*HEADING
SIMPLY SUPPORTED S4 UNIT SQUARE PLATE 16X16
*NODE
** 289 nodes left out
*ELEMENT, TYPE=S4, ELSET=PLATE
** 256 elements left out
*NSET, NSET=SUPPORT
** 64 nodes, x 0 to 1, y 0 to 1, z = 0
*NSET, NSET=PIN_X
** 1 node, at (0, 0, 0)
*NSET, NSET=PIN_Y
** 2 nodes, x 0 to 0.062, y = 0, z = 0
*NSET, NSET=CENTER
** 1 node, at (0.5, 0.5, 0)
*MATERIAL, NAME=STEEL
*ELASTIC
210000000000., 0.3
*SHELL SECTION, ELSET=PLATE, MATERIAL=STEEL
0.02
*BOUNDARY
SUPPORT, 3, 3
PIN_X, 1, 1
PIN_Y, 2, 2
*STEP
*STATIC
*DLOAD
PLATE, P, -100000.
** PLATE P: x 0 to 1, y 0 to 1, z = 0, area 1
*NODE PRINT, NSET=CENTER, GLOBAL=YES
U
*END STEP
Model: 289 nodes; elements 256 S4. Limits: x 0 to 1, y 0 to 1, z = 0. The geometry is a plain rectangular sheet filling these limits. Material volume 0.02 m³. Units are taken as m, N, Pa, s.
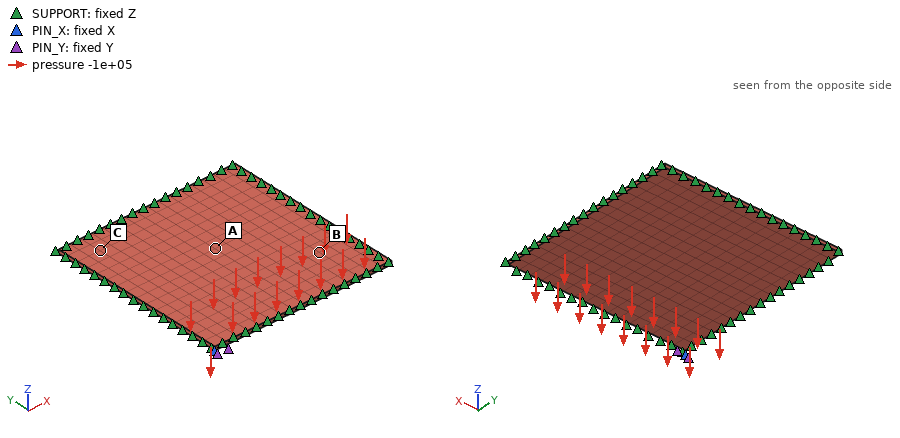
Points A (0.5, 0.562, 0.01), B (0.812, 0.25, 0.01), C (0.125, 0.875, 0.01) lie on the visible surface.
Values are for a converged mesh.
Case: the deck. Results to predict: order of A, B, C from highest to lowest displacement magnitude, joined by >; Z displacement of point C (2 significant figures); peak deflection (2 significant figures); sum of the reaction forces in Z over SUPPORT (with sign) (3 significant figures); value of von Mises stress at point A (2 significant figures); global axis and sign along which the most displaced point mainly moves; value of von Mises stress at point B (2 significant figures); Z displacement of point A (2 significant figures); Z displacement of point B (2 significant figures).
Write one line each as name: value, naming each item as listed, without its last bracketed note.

order of A, B, C from highest to lowest displacement magnitude, joined by >: A > B > C
Z displacement of point C: -4.4e-04 m
peak deflection: 0.0027 m
sum of the reaction forces in Z over SUPPORT (with sign): 1.00e+05 N
value of von Mises stress at point A: 7.2e+07 Pa
global axis and sign along which the most displaced point mainly moves: -Z
value of von Mises stress at point B: 5.7e+07 Pa
Z displacement of point A: -0.0026 m
Z displacement of point B: -0.0011 m
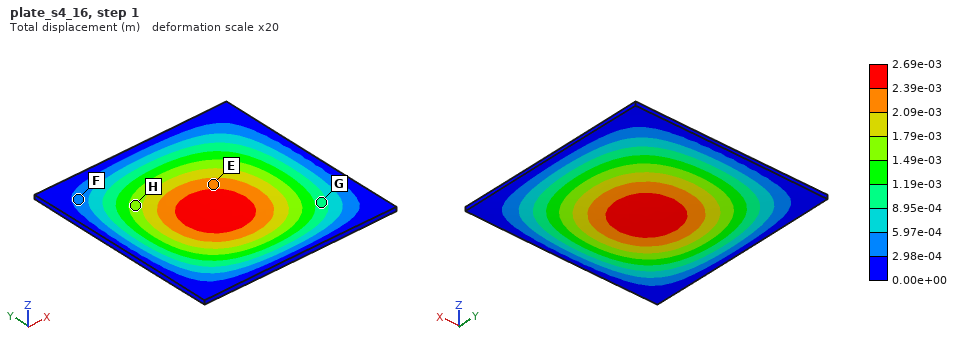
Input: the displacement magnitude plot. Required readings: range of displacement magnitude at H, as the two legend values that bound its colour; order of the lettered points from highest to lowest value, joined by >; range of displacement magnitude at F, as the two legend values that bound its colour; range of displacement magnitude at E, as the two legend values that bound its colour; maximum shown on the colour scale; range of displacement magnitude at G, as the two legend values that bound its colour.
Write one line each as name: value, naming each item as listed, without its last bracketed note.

range of displacement magnitude at H, as the two legend values that bound its colour: 1.49e-03 to 1.79e-03 m
order of the lettered points from highest to lowest value, joined by >: E > H > G > F
range of displacement magnitude at F, as the two legend values that bound its colour: 2.98e-04 to 5.97e-04 m
range of displacement magnitude at E, as the two legend values that bound its colour: 2.09e-03 to 2.39e-03 m
maximum shown on the colour scale: 2.69e-03 m
range of displacement magnitude at G, as the two legend values that bound its colour: 8.95e-04 to 1.19e-03 m
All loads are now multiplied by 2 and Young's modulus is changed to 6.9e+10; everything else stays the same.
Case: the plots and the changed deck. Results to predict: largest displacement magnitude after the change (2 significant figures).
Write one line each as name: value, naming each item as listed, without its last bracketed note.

largest displacement magnitude after the change: 0.016 m
